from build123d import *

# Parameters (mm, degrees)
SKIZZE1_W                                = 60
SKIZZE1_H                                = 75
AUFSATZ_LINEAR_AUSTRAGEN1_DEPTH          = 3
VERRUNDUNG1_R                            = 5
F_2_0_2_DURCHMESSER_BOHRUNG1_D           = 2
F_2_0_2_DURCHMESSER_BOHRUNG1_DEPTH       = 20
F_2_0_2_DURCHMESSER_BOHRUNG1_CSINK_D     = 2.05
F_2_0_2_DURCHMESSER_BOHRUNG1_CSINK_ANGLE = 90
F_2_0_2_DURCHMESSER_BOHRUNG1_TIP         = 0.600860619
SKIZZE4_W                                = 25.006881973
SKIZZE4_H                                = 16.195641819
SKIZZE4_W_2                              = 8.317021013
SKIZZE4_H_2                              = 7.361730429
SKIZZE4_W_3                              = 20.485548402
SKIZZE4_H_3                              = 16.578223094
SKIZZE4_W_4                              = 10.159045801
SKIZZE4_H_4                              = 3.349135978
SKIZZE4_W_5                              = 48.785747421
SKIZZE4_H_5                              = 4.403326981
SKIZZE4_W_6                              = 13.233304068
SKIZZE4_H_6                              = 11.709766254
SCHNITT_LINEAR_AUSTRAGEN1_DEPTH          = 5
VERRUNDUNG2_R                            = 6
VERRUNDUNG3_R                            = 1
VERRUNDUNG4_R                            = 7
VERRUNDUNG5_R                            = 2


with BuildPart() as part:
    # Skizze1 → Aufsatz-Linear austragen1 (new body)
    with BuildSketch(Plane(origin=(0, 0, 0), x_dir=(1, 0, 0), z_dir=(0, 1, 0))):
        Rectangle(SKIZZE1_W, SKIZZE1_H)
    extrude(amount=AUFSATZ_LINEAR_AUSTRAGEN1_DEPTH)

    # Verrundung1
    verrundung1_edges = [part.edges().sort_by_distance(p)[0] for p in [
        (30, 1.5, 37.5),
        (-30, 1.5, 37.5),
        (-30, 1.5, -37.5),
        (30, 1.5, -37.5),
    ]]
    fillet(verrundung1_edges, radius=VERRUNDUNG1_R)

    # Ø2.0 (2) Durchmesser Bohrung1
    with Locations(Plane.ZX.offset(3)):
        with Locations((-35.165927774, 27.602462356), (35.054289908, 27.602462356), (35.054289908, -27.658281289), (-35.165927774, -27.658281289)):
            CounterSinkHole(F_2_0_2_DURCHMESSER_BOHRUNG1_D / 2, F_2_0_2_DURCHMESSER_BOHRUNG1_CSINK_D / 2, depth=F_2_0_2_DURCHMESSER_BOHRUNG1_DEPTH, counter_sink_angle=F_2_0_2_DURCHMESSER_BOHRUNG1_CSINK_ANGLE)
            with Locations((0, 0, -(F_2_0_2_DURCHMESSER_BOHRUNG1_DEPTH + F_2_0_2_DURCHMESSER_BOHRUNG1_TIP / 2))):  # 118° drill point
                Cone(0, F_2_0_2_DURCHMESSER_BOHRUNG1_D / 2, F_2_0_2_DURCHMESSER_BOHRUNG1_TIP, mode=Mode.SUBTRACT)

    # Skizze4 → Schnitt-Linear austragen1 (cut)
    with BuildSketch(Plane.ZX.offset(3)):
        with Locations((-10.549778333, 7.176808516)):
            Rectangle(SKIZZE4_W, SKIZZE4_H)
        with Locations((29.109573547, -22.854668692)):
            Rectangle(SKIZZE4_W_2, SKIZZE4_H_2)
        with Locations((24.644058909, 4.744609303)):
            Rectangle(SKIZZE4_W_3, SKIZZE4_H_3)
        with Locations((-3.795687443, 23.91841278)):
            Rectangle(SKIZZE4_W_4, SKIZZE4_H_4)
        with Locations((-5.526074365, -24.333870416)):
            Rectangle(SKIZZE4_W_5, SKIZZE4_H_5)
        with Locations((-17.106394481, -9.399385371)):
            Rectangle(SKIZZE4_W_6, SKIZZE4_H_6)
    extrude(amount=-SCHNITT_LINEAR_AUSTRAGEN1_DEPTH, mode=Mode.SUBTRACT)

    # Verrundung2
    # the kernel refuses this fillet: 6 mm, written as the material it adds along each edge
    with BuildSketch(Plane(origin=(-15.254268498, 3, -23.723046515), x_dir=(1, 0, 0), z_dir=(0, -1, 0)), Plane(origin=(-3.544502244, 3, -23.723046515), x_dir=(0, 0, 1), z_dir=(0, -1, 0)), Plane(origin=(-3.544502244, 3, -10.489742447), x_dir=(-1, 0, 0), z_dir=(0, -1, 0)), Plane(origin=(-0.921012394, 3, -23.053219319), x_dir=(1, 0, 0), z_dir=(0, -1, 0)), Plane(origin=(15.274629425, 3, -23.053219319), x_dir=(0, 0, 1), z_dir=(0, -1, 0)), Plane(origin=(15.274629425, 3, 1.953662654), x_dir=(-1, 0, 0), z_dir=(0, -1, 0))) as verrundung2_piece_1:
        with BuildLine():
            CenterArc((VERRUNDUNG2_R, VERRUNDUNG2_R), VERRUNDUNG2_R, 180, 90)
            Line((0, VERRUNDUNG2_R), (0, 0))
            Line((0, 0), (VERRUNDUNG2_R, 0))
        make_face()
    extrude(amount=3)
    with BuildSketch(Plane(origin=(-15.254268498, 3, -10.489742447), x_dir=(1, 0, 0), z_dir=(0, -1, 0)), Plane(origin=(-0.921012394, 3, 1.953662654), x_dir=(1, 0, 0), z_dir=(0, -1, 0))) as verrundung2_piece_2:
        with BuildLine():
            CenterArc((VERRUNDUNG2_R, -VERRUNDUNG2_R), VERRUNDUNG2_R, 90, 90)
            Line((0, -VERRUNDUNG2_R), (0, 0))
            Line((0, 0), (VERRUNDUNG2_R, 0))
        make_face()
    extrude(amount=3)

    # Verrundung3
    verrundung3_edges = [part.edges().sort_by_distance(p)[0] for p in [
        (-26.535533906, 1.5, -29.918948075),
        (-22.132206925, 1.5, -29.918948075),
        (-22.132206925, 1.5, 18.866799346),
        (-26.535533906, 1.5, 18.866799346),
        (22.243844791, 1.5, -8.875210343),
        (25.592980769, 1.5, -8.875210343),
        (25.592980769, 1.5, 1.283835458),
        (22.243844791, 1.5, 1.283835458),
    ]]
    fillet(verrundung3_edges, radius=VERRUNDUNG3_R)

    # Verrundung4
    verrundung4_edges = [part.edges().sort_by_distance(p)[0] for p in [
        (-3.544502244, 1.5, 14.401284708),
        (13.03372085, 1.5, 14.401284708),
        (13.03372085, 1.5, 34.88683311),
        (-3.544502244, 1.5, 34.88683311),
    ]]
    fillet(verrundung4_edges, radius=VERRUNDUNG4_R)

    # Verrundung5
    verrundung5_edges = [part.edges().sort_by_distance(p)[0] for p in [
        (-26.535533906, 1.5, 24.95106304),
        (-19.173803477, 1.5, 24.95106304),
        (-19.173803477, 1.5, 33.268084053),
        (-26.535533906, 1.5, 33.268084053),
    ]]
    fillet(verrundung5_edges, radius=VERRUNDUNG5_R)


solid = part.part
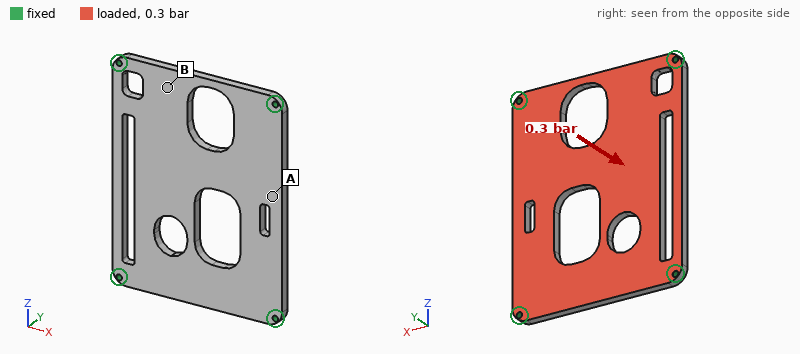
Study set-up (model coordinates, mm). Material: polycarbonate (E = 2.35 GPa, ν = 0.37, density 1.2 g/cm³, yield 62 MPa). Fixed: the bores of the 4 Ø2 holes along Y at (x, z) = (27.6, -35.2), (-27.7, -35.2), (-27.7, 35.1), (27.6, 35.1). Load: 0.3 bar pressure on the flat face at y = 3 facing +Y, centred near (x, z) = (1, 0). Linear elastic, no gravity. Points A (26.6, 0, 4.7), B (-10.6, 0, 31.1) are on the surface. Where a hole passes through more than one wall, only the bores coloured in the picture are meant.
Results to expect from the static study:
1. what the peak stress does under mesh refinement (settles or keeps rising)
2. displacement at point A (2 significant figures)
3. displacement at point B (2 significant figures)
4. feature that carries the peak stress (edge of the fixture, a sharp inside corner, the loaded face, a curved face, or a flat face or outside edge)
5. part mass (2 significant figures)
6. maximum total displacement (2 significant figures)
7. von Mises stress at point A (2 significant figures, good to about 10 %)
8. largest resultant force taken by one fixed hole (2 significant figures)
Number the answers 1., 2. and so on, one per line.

1. keeps rising
2. 0.64 mm
3. 0.35 mm
4. edge of the fixture
5. 12 g
6. 1.0 mm
7. 5.4 MPa
8. 27 N
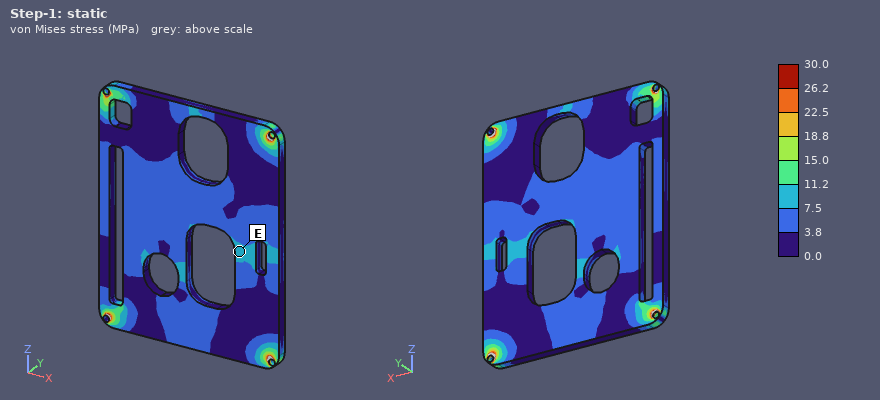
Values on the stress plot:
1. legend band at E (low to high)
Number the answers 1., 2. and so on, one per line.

1. 7.5 to 11.2 MPa
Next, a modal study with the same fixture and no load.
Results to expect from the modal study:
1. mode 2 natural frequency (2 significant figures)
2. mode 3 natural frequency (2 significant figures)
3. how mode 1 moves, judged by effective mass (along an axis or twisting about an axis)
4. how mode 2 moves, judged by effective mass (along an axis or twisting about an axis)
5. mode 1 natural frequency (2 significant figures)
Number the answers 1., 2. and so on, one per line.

1. 940 Hz
2. 1200 Hz
3. along Y
4. twisting about Z
5. 560 Hz
